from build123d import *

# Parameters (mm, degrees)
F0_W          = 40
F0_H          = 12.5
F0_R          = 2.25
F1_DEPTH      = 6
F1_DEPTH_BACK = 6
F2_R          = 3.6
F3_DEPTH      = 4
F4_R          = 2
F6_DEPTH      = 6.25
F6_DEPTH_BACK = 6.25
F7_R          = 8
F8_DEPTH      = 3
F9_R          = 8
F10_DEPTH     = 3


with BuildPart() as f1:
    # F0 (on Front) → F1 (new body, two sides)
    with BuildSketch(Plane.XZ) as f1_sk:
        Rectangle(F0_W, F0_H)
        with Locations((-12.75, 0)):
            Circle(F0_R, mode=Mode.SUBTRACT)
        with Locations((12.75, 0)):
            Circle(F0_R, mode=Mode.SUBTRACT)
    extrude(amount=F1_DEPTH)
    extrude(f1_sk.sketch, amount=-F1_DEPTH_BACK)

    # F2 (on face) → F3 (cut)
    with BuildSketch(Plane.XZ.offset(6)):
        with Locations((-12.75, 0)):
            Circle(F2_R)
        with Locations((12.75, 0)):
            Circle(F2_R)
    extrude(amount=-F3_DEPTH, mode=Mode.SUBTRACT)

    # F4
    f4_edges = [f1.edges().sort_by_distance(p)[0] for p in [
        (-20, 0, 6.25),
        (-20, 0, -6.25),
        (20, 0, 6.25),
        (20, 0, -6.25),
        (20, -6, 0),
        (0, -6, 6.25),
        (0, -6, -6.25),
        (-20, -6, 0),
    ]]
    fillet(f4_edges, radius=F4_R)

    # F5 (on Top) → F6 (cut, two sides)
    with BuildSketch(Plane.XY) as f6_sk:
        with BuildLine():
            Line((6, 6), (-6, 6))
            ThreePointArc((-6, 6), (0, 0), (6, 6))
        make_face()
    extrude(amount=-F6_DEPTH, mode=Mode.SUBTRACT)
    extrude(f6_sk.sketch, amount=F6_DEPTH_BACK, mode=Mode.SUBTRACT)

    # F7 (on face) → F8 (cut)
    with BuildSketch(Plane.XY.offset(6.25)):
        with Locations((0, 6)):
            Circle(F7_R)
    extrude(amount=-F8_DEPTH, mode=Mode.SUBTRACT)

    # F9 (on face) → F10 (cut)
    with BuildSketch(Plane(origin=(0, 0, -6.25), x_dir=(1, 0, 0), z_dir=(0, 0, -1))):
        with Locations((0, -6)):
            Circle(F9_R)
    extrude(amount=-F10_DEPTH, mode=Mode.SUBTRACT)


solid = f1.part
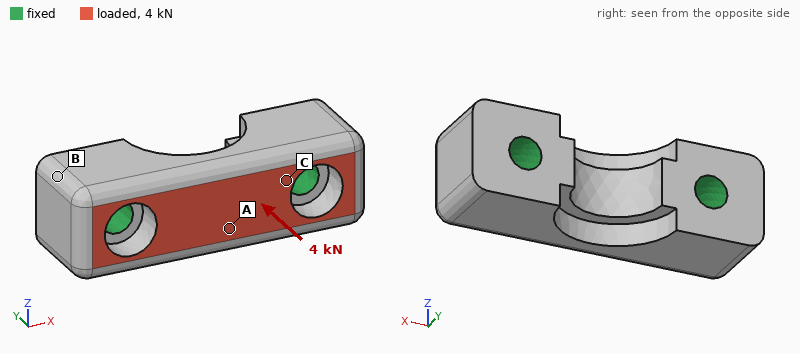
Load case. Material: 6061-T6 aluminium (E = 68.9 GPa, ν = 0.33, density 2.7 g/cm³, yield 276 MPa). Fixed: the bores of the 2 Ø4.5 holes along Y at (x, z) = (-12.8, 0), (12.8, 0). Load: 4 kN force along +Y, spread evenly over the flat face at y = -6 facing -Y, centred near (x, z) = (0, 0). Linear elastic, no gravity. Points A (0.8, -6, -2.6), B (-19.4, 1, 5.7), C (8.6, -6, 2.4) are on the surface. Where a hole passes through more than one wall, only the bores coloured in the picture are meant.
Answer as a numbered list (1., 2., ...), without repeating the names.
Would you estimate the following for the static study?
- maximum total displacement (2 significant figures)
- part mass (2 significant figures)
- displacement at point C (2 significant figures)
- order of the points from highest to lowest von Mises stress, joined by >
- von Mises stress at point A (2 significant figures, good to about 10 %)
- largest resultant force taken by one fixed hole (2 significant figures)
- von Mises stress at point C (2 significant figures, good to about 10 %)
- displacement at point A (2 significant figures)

1. 7.9 µm
2. 12 g
3. 4.4 µm
4. A > C > B
5. 25 MPa
6. 2.2 kN
7. 15 MPa
8. 7.8 µm
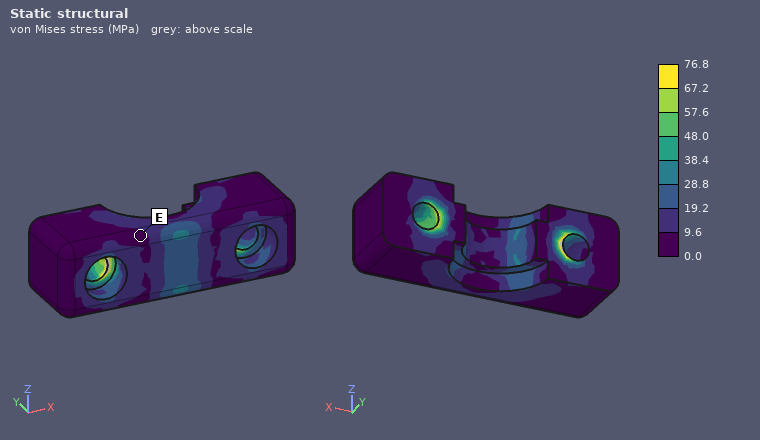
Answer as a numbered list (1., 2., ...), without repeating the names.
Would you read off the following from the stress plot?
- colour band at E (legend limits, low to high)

1. 0.0 to 9.6 MPa
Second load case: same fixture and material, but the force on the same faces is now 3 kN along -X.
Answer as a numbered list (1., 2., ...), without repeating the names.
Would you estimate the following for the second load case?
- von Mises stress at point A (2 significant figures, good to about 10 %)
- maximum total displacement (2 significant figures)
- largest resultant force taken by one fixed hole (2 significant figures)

1. 25 MPa
2. 5.3 µm
3. 1.6 kN
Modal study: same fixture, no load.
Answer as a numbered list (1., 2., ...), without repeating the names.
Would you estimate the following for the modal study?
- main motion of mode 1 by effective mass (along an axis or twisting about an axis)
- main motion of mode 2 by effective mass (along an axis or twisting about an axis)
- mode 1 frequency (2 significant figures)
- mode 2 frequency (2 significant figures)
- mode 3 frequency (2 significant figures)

1. along Z
2. along Y
3. 38 kHz
4. 53 kHz
5. 57 kHz
